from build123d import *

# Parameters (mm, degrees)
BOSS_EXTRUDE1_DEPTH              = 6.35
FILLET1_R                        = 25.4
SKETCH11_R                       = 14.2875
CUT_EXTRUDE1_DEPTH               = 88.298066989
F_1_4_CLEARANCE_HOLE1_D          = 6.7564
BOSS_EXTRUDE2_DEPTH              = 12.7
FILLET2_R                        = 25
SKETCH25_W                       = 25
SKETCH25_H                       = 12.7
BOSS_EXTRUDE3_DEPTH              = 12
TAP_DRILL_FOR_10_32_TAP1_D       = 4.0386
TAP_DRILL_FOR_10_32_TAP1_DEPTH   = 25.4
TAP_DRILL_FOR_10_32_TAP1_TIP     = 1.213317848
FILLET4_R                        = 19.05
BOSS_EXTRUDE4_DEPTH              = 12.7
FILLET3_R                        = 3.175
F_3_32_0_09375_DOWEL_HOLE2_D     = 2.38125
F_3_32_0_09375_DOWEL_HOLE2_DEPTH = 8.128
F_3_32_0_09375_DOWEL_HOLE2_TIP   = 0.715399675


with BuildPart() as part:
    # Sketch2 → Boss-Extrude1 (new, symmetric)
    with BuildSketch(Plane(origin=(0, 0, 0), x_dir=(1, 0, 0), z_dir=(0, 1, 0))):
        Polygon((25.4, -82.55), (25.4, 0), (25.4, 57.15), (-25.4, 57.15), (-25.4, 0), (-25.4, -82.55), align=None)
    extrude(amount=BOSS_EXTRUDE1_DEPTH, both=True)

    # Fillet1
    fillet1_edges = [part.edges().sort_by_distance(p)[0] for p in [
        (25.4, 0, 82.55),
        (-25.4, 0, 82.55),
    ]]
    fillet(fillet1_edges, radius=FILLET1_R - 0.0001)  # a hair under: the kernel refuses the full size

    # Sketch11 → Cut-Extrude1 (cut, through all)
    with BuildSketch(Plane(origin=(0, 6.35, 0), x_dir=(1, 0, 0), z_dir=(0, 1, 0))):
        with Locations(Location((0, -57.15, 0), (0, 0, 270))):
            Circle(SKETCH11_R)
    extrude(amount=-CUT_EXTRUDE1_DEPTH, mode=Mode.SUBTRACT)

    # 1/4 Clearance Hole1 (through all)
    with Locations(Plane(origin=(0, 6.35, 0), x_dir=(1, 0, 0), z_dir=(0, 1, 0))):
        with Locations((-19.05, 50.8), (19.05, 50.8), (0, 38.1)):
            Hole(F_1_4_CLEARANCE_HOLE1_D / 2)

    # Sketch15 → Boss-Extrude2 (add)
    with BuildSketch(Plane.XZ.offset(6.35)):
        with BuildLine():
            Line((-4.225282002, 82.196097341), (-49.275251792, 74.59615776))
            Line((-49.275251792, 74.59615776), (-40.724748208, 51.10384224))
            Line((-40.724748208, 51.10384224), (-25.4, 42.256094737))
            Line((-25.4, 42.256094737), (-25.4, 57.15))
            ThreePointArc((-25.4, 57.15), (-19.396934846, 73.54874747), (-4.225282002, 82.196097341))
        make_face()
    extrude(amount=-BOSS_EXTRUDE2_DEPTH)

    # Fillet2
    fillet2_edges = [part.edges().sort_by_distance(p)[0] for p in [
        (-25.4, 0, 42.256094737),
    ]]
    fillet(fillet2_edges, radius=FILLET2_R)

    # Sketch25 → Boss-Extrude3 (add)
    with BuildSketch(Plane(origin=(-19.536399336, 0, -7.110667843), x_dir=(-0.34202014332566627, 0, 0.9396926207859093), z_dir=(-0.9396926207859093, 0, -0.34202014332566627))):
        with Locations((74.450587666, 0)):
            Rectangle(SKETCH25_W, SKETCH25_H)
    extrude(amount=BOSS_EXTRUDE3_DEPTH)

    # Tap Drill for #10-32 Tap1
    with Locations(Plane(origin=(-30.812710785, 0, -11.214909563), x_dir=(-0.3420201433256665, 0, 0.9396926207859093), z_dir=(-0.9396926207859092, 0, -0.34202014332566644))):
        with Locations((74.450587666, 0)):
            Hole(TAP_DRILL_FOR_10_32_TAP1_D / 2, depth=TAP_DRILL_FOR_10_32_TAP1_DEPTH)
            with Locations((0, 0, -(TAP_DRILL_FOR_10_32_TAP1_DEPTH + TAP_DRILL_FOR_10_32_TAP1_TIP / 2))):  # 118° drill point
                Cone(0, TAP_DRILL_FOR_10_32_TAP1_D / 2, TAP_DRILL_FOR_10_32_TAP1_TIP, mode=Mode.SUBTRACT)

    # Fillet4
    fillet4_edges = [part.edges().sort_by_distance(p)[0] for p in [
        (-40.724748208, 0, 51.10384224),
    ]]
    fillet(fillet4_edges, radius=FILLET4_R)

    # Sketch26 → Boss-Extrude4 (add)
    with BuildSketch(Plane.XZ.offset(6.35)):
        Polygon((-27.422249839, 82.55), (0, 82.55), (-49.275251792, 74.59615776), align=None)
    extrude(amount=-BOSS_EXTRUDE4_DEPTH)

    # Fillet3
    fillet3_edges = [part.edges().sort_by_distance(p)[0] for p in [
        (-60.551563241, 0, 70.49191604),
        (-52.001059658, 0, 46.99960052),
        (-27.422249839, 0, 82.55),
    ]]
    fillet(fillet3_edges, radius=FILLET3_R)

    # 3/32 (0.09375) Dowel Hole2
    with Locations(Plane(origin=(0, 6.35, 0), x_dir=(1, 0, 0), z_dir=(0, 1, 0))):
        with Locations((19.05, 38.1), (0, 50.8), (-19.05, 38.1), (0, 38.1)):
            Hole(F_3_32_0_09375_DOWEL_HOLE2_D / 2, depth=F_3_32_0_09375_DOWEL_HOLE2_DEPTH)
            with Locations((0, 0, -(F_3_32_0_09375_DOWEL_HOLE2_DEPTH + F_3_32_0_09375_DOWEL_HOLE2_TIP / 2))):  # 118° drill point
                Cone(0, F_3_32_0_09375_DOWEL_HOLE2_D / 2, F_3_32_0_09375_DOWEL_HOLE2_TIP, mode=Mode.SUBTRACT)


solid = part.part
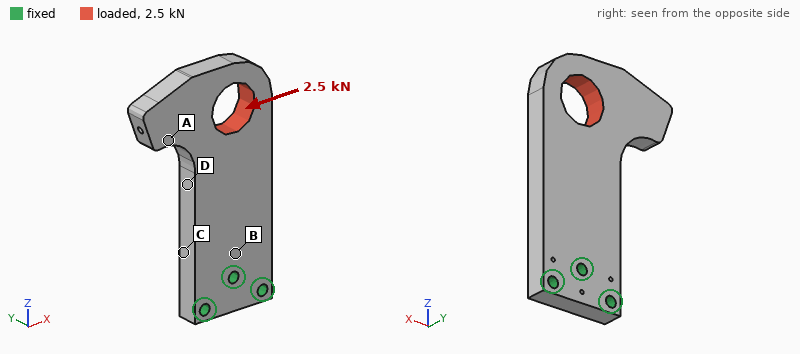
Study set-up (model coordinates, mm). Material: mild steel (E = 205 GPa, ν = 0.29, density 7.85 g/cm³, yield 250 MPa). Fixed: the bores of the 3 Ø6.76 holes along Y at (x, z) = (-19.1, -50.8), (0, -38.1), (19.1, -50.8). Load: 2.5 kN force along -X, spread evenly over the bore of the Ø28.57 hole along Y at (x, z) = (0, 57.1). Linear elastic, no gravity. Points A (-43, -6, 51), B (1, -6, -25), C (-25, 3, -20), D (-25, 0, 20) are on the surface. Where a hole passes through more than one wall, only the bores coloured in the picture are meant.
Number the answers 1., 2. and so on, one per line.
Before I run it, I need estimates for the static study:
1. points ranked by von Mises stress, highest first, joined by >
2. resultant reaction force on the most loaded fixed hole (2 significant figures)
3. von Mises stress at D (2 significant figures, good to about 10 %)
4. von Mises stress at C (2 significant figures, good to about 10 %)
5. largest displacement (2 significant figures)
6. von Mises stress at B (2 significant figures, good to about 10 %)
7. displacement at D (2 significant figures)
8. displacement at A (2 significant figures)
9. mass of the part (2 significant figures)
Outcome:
1. C > D > B > A
2. 5.5 kN
3. 19 MPa
4. 36 MPa
5. 61 µm
6. 10 MPa
7. 23 µm
8. 45 µm
9. 710 g
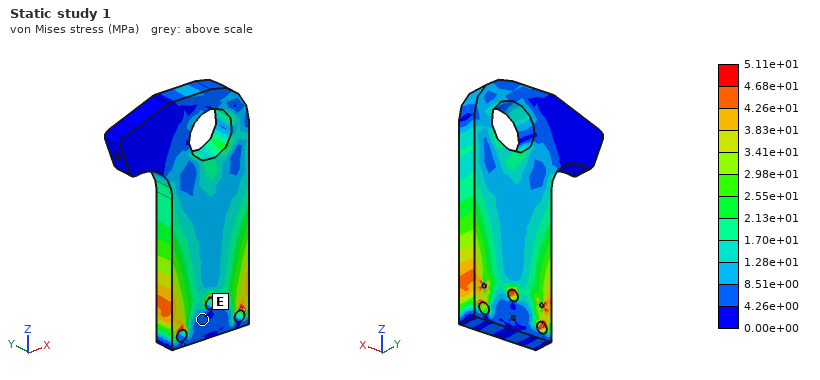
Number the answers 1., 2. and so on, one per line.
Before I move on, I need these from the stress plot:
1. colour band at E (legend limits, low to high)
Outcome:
1. 4.26e+00 to 8.51e+00 MPa
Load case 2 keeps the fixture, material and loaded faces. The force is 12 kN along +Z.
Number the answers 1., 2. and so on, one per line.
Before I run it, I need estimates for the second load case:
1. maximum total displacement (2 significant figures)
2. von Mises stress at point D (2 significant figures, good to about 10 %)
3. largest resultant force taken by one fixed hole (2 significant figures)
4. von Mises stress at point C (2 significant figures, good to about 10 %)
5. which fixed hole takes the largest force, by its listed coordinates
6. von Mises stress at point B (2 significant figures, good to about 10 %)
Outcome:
1. 15 µm
2. 24 MPa
3. 6.2 kN
4. 15 MPa
5. (0, -38.1)
6. 25 MPa
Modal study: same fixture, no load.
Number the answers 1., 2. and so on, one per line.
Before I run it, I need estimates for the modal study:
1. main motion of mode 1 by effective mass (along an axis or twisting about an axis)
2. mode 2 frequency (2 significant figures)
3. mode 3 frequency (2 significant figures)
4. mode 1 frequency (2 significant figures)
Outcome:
1. along Y
2. 2000 Hz
3. 2000 Hz
4. 650 Hz
